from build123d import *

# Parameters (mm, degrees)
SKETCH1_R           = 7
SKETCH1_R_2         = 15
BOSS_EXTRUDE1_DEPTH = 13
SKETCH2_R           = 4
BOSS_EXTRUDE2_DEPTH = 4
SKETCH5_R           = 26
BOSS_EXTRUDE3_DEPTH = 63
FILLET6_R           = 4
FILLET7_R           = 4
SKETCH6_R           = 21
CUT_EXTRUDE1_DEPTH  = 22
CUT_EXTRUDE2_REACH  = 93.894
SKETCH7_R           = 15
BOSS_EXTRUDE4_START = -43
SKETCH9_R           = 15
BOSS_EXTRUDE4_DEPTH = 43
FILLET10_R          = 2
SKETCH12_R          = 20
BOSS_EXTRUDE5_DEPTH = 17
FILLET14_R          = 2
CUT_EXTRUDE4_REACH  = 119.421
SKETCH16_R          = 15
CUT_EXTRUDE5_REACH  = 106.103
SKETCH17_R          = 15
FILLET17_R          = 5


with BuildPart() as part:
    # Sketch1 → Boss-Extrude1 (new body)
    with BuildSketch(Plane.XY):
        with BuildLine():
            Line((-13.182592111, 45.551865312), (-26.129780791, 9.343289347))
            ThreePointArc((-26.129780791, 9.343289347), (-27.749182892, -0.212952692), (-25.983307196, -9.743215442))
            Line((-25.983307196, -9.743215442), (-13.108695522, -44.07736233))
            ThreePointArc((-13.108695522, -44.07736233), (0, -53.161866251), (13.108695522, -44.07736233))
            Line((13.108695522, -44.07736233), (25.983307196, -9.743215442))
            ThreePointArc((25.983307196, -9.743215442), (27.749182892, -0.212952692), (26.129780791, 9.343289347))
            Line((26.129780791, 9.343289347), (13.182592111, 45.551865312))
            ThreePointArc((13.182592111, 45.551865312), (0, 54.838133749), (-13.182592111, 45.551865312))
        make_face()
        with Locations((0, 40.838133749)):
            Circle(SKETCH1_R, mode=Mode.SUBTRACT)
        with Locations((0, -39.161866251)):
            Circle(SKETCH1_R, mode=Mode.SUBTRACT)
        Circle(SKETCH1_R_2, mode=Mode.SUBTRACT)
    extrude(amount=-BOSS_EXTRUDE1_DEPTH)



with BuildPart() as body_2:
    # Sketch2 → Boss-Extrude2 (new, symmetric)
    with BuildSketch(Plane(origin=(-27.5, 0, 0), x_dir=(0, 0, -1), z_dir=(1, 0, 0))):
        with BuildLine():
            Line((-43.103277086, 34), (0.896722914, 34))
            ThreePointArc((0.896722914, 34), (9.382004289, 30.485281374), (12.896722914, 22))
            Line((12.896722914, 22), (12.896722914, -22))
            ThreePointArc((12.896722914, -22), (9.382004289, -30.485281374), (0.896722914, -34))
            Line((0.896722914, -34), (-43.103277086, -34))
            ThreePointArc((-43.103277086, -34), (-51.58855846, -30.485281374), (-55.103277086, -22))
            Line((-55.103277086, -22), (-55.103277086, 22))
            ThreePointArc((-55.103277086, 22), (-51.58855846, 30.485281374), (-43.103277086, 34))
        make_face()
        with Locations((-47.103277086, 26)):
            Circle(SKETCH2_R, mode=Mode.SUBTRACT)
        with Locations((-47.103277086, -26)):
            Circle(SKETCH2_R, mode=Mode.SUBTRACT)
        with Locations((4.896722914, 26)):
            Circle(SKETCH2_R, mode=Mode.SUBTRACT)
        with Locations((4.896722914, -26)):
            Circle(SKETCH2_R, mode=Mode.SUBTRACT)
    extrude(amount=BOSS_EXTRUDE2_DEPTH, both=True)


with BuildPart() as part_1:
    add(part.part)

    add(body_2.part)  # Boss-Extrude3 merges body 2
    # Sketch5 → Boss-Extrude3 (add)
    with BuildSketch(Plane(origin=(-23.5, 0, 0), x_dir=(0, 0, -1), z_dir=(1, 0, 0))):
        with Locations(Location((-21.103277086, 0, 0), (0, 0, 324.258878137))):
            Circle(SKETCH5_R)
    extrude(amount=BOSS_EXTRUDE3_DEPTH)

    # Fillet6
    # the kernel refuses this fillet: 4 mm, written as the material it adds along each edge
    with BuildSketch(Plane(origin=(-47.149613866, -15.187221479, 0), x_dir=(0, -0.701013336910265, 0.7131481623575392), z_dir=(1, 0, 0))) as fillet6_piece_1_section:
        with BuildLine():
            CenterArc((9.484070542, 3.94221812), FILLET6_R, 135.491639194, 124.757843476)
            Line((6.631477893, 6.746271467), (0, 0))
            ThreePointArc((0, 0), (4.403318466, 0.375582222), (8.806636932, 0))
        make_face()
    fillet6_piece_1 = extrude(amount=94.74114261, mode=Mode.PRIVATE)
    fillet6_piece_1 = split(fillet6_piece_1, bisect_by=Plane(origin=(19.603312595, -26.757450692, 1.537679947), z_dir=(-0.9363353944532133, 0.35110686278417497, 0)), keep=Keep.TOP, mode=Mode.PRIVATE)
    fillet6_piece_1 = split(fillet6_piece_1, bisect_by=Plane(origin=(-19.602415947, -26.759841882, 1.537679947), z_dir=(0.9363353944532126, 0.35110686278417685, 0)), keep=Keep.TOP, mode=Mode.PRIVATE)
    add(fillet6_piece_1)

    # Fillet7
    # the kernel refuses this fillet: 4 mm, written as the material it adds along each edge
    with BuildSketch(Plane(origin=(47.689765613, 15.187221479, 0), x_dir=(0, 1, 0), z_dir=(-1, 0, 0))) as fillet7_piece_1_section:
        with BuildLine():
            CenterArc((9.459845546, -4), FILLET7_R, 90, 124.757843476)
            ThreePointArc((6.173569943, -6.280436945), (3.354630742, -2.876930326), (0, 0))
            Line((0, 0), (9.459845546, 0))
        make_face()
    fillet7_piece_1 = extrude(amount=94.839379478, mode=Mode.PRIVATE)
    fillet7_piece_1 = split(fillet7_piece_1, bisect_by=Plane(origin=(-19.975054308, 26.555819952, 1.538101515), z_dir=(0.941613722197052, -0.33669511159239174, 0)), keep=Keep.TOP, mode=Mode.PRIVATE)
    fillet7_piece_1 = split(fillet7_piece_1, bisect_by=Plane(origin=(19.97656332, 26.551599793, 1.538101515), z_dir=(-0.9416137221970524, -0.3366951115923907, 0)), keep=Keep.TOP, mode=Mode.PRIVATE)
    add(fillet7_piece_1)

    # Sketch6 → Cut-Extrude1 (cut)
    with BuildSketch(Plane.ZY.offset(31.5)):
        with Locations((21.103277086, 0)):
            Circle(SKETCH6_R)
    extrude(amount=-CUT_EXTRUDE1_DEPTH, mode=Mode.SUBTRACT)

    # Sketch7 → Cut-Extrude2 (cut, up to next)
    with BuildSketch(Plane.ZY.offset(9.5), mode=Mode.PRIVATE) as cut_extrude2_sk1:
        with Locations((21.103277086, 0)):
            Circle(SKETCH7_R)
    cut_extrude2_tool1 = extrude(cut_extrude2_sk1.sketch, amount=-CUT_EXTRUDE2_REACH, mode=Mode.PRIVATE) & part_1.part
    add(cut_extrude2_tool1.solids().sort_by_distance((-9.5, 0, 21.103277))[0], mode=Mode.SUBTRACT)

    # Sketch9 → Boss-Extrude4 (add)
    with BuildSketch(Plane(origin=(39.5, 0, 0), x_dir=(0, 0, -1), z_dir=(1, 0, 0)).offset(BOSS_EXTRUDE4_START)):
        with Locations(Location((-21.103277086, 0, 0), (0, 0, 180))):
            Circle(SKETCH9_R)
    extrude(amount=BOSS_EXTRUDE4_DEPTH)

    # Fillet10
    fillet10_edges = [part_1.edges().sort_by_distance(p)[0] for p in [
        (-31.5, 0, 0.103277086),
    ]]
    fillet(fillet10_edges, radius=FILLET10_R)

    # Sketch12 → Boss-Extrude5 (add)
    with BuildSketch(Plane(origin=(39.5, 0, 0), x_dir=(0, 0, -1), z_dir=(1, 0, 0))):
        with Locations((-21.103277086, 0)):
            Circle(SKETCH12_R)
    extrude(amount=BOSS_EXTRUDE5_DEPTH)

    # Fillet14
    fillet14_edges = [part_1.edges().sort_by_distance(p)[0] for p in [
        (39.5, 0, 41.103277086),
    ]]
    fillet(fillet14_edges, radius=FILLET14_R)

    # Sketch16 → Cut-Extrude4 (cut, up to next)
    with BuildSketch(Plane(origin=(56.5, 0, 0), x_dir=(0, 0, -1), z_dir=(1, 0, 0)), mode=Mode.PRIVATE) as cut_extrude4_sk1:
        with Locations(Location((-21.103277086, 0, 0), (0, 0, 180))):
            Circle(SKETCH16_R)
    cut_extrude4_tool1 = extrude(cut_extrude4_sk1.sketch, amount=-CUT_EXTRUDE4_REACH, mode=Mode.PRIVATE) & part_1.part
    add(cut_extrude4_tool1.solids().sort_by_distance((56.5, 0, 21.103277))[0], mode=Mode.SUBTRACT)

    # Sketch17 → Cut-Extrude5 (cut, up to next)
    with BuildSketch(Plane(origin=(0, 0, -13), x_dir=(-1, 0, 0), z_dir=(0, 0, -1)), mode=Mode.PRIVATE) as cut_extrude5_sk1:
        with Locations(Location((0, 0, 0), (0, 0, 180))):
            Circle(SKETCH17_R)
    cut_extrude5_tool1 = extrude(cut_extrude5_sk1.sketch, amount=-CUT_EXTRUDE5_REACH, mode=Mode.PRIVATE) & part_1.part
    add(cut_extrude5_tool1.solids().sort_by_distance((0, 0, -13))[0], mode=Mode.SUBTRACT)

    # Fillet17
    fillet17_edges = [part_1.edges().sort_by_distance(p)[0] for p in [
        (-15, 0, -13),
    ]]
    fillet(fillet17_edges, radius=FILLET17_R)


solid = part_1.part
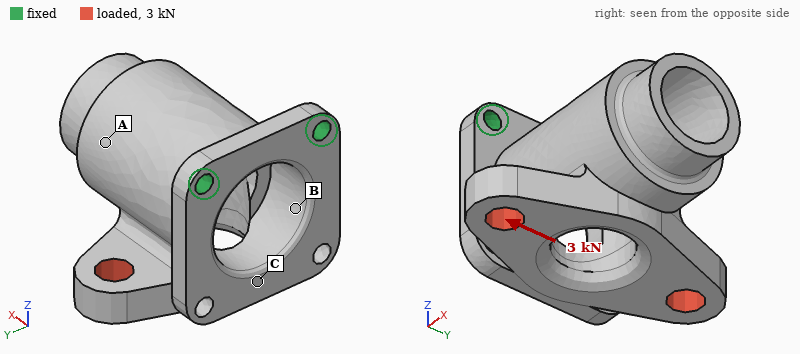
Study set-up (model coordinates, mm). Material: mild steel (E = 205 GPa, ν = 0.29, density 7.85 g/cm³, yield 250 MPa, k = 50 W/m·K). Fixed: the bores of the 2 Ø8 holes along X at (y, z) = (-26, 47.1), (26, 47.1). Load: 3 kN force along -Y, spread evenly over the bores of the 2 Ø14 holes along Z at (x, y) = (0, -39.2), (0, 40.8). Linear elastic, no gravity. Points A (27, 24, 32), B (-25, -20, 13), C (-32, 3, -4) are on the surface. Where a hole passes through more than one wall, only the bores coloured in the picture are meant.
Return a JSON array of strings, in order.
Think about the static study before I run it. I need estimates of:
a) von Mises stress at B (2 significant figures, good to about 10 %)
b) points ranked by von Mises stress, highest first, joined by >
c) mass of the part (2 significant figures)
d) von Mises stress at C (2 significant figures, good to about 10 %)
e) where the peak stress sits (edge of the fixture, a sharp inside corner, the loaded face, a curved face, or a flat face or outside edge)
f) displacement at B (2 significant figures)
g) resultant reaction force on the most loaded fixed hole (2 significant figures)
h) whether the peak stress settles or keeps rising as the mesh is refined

["32 MPa", "B > C > A", "1.1 kg", "16 MPa", "edge of the fixture", "12 µm", "3.5 kN", "keeps rising"]
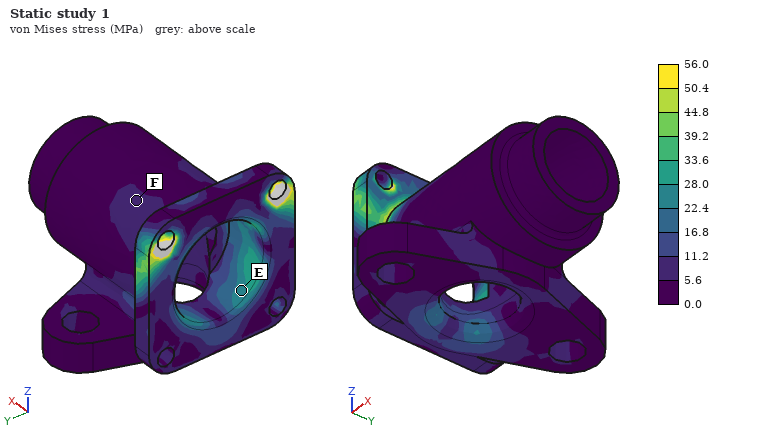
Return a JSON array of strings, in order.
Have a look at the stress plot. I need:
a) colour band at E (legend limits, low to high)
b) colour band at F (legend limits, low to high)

["22.4 to 28.0 MPa", "5.6 to 11.2 MPa"]
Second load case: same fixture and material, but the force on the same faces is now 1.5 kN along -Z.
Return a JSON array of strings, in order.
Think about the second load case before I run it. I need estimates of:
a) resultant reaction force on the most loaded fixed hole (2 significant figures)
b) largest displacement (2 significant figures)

["780 N", "94 µm"]
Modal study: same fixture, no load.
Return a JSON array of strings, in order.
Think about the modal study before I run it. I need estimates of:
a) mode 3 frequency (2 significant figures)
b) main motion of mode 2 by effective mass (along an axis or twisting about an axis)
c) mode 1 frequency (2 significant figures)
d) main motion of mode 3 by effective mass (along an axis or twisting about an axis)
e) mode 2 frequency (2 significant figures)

["3100 Hz", "along Y", "590 Hz", "along Y", "1800 Hz"]
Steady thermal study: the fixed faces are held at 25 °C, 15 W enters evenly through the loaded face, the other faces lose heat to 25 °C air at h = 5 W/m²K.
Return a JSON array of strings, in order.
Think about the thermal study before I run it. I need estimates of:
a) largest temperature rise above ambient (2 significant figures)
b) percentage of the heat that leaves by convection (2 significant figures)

["32 K", "21 %"]
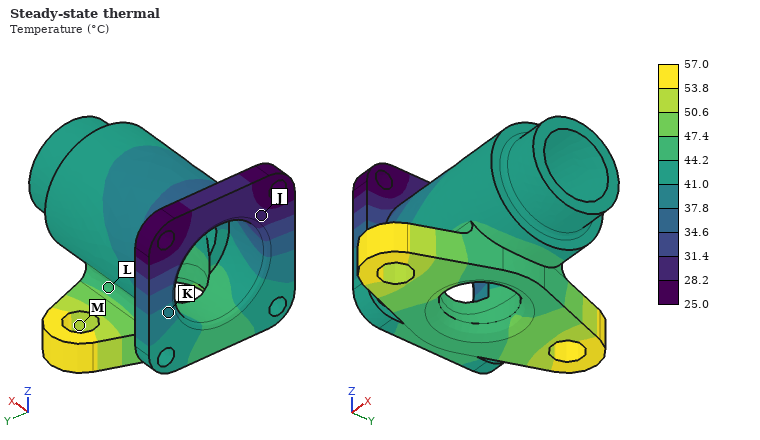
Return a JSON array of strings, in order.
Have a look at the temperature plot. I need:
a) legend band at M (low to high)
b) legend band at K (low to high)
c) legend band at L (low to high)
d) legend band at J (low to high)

["50.6 to 53.8 °C", "37.8 to 41.0 °C", "44.2 to 47.4 °C", "28.2 to 31.4 °C"]
